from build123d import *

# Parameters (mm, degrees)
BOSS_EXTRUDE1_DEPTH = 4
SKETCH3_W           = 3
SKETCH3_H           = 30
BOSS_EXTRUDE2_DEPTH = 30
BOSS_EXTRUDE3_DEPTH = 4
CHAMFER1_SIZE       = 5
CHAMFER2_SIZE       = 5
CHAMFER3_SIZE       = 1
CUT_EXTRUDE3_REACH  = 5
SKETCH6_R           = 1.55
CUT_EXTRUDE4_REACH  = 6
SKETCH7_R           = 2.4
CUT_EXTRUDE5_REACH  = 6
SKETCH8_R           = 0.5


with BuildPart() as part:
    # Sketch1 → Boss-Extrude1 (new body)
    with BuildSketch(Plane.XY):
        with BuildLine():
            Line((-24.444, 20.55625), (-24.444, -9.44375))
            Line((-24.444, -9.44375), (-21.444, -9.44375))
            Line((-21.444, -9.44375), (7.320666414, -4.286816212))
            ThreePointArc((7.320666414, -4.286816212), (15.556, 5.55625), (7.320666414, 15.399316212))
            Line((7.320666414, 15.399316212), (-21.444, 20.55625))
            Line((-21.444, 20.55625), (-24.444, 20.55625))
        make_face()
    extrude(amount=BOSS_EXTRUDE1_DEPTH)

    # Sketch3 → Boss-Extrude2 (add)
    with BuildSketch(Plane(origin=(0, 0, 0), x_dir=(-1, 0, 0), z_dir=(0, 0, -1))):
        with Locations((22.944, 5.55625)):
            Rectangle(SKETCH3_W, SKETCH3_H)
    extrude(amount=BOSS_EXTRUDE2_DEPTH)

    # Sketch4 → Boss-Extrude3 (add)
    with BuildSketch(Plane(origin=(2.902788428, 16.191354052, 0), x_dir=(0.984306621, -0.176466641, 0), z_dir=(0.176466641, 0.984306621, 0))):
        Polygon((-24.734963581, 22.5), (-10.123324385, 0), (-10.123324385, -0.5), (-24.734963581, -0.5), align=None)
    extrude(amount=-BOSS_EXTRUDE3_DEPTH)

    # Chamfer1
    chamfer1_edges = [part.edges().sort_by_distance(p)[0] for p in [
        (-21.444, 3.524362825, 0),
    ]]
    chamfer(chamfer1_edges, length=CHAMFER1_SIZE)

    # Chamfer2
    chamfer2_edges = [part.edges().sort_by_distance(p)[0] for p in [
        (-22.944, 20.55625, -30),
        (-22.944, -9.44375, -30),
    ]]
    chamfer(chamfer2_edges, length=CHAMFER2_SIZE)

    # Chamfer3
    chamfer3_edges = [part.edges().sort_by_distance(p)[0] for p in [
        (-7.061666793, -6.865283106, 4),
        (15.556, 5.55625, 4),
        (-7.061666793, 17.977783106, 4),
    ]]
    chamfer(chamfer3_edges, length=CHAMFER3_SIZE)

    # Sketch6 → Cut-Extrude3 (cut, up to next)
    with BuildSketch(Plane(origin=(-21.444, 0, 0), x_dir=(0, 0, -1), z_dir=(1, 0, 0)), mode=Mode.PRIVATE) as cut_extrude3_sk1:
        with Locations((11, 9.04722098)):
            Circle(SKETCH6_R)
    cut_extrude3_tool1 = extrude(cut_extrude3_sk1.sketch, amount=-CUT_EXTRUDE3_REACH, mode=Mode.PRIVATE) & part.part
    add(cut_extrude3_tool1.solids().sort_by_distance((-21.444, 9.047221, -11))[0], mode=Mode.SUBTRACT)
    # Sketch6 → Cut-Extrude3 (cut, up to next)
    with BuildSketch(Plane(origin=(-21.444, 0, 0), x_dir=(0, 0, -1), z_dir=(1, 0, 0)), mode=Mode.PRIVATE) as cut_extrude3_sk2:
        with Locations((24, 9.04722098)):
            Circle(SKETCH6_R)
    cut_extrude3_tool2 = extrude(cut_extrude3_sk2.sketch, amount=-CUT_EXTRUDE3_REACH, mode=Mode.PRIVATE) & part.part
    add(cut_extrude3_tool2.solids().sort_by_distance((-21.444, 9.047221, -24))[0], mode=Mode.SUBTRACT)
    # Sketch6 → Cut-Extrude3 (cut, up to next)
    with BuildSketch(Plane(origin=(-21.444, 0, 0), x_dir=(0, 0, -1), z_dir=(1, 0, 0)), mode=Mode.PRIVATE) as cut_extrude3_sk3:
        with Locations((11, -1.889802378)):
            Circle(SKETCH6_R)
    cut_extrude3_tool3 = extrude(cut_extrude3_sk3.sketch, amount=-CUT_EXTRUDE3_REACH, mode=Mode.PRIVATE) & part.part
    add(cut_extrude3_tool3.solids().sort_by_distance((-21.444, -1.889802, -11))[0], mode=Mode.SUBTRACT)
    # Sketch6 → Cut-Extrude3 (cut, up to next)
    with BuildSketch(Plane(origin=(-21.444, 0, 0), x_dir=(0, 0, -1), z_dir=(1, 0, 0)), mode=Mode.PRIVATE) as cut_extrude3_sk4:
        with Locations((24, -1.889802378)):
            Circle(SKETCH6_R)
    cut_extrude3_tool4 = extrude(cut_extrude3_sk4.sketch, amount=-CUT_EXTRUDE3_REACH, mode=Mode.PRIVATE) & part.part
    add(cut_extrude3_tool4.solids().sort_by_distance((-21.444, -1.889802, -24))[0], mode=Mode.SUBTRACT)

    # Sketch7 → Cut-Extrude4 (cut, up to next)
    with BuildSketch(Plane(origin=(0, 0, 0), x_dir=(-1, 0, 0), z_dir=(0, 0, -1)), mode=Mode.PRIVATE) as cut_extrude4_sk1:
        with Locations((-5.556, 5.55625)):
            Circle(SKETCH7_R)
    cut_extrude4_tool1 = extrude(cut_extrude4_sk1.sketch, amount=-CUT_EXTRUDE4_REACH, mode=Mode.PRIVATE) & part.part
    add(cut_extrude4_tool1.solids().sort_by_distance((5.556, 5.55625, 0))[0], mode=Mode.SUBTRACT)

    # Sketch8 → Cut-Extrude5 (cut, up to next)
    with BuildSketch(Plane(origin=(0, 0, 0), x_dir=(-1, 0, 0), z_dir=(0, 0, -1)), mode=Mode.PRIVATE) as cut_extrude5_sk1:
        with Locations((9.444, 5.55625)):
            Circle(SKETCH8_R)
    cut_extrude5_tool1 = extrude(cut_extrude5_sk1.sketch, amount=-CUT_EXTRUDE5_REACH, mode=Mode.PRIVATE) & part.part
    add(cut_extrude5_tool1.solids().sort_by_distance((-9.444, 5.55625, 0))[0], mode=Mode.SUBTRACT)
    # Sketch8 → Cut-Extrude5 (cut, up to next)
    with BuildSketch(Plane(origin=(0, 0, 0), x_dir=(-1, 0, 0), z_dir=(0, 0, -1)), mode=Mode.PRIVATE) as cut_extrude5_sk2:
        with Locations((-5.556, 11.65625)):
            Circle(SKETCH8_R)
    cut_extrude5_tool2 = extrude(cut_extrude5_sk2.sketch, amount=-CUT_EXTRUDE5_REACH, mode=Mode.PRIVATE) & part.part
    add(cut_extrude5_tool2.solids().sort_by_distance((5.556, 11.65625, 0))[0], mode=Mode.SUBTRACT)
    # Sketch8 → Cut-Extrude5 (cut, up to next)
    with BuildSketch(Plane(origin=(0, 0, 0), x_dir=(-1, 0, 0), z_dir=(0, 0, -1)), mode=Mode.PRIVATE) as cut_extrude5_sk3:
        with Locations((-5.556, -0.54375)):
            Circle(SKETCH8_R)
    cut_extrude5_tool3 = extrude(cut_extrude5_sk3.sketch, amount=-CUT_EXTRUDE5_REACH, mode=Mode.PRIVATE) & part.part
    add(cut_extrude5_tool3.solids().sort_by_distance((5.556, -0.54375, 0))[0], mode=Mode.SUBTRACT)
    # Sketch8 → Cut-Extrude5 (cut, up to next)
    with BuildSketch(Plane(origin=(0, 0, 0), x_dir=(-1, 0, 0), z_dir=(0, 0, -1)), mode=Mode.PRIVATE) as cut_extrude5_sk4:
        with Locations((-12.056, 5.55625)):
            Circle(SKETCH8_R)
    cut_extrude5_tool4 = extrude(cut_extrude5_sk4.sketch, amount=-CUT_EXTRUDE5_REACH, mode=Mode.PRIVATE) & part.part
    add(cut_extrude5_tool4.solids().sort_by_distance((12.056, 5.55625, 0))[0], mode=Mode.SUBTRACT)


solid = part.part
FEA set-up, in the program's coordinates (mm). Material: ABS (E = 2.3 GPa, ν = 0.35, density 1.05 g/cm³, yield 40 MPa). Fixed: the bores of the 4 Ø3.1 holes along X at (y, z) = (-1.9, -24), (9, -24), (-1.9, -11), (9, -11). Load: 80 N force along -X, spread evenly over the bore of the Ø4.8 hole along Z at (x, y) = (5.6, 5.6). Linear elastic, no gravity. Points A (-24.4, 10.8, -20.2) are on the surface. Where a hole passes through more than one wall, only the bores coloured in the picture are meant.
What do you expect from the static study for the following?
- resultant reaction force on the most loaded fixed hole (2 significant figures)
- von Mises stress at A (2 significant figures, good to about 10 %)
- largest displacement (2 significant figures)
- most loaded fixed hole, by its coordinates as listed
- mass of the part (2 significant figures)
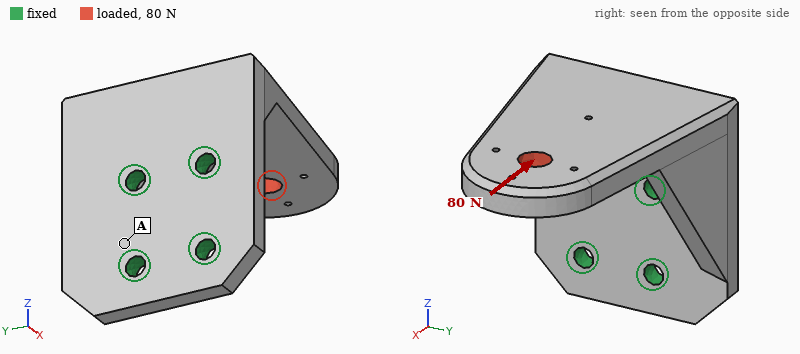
89 N
3.2 MPa
0.70 mm
(9, -11)
7.4 g
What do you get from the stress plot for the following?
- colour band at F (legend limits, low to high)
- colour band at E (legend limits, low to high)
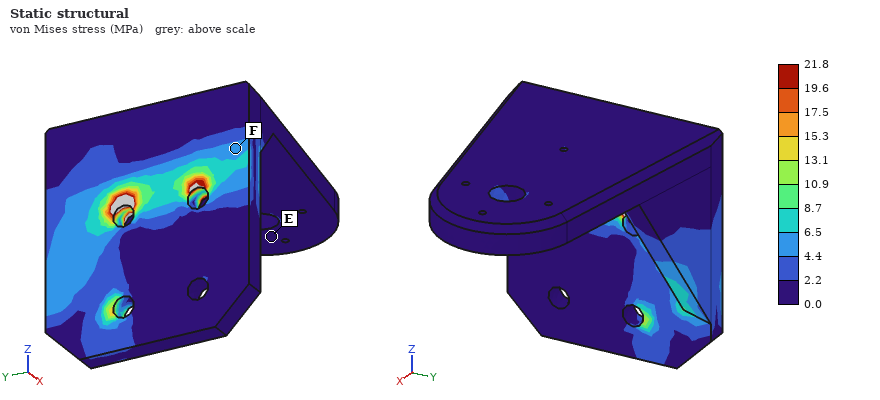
4.4 to 6.5 MPa
0.0 to 2.2 MPa
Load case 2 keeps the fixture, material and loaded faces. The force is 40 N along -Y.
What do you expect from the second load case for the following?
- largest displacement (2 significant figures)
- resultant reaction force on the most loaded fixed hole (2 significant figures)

0.54 mm
82 N
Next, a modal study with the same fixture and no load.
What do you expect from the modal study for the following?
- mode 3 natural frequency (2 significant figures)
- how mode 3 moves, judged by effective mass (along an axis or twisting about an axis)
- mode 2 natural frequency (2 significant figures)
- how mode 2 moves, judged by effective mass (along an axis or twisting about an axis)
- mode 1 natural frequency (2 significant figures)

2200 Hz
along X
1200 Hz
along Y
720 Hz
